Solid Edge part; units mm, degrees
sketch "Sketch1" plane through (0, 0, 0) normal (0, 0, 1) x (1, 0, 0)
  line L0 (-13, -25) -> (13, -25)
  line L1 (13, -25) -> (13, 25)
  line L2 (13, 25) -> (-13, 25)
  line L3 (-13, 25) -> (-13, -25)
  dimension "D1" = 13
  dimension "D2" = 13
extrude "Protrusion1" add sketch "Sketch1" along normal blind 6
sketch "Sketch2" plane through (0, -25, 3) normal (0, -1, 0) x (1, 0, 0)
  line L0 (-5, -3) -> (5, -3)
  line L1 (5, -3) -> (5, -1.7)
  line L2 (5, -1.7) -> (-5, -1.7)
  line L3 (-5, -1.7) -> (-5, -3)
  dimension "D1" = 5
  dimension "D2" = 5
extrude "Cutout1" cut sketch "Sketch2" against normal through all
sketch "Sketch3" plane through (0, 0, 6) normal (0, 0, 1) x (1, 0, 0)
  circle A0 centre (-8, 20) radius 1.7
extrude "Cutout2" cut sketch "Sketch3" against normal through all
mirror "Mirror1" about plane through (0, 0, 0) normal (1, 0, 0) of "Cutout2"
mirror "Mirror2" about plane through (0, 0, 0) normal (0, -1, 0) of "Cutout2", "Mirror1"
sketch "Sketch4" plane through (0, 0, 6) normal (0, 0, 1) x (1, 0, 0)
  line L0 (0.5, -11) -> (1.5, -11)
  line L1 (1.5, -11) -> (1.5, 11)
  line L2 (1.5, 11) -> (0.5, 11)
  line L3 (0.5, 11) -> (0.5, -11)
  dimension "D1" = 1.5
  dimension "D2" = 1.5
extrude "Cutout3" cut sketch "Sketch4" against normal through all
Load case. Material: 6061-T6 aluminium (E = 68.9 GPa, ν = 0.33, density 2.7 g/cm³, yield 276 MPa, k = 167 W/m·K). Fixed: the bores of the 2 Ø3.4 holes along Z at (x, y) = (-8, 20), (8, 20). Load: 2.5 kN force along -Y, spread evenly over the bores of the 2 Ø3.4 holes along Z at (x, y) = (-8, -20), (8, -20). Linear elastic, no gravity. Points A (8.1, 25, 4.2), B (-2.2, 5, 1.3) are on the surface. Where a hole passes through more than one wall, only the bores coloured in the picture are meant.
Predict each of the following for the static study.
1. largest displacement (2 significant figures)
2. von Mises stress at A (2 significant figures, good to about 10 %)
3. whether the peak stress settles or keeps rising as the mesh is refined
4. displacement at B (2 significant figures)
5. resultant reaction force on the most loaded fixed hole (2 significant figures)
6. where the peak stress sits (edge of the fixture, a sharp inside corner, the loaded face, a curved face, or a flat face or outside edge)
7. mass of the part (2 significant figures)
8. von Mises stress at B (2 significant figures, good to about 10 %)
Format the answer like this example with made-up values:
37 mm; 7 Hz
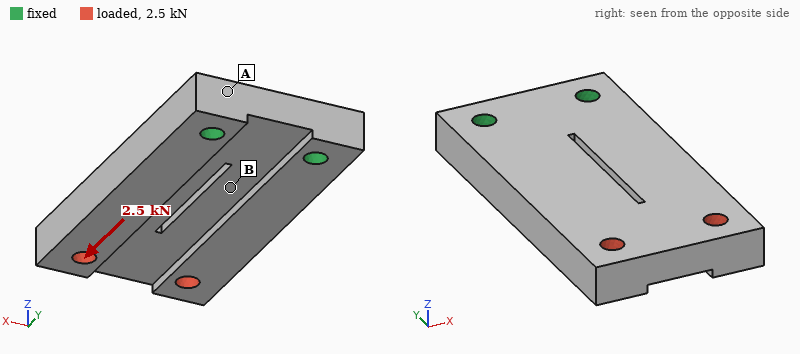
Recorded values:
22 µm; 10 MPa; keeps rising; 4.9 µm; 1.3 kN; edge of the fixture; 18 g; 20 MPa
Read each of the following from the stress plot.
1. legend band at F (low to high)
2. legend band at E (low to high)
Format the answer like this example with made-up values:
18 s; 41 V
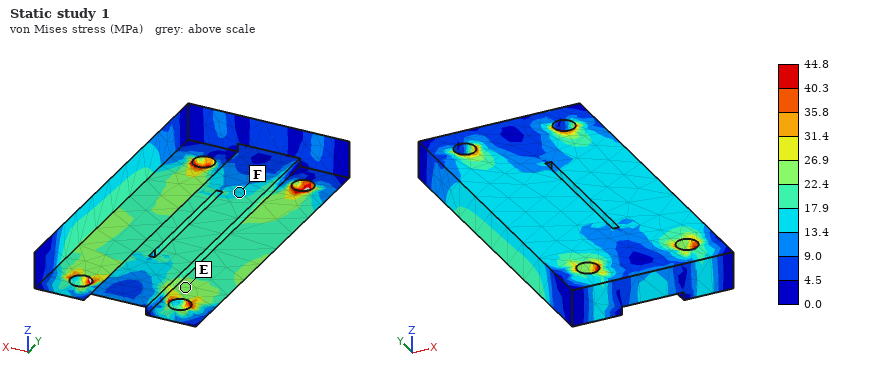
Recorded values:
13.4 to 17.9 MPa; 22.4 to 26.9 MPa
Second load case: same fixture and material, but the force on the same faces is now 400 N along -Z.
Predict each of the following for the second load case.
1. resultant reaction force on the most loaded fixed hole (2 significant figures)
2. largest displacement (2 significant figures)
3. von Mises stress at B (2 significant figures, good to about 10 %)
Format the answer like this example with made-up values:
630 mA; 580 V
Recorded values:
220 N; 0.38 mm; 53 MPa
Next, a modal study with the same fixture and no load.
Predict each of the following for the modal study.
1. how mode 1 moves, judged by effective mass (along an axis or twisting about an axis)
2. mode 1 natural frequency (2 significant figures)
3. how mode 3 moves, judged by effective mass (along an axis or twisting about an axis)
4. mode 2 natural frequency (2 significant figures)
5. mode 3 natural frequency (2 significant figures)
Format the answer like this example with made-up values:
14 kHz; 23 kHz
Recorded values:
along Z; 2400 Hz; along X; 7000 Hz; 7700 Hz
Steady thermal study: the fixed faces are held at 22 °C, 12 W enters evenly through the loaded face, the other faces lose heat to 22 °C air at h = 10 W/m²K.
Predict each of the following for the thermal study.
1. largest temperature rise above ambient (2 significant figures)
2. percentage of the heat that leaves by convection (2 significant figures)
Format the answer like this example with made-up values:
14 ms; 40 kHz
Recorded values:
21 K; 3.1 %
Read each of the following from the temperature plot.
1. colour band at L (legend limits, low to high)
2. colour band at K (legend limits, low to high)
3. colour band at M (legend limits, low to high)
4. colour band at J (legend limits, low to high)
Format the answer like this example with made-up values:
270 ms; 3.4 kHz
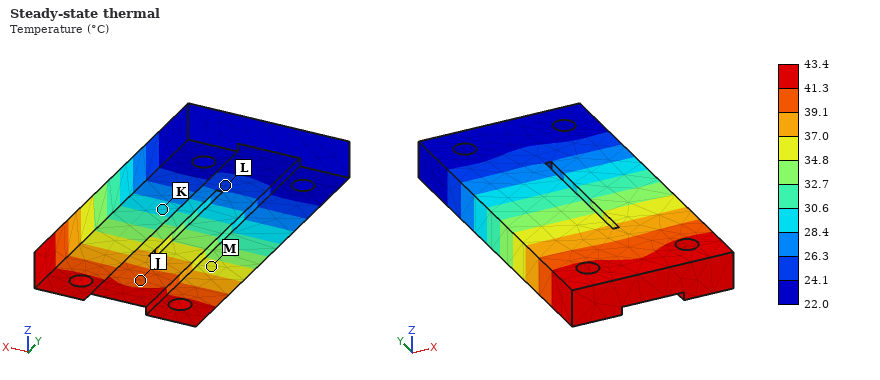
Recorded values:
24.1 to 26.3 °C; 28.4 to 30.6 °C; 34.8 to 37.0 °C; 39.1 to 41.3 °C
